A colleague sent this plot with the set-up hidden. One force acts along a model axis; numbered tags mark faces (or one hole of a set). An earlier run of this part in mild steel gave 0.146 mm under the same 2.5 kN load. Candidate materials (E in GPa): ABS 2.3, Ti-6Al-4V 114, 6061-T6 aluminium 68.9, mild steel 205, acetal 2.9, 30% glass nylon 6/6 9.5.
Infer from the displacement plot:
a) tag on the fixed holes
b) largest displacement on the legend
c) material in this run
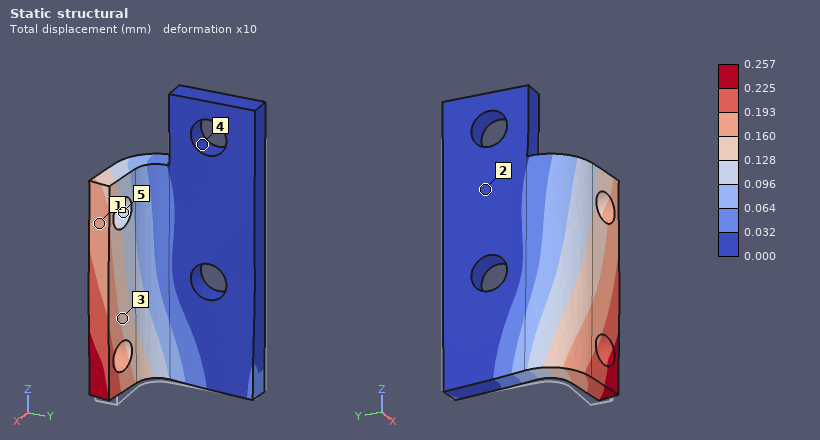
4
0.257 mm
Ti-6Al-4V
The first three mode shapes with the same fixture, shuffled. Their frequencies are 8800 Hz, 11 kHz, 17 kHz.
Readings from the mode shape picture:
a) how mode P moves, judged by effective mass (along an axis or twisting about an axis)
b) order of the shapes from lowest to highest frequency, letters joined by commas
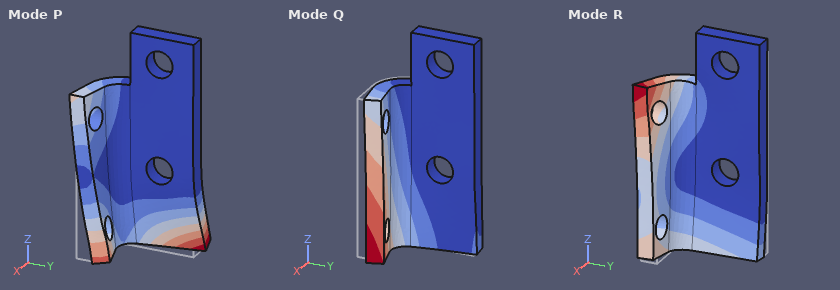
along X
Q, R, P
